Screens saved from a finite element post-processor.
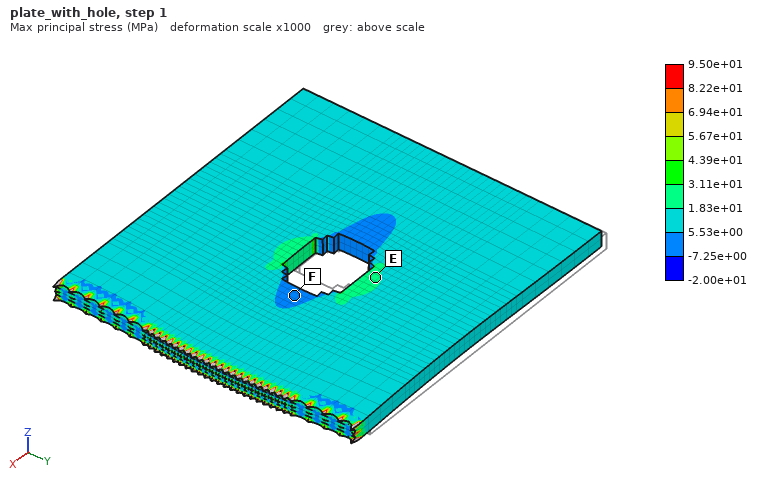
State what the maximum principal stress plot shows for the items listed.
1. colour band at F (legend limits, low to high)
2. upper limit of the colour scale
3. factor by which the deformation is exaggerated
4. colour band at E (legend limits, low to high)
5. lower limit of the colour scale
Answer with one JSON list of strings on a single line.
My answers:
["-7.25e+00 to 5.53e+00 MPa", "9.50e+01 MPa", "1000", "1.83e+01 to 3.11e+01 MPa", "-2.00e+01 MPa"]
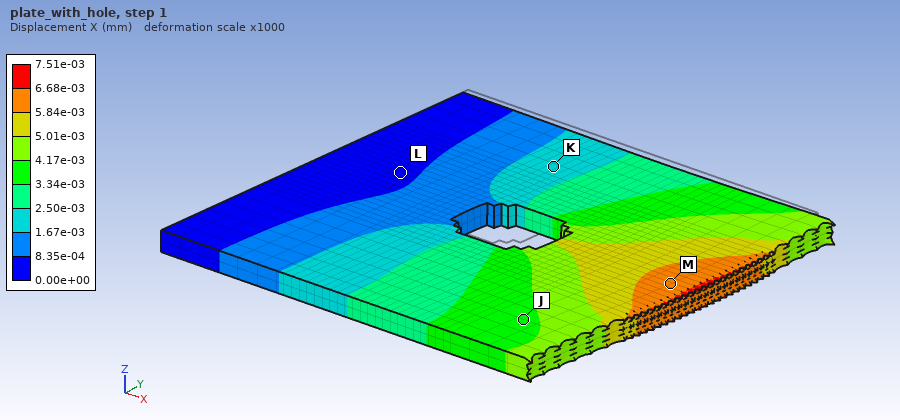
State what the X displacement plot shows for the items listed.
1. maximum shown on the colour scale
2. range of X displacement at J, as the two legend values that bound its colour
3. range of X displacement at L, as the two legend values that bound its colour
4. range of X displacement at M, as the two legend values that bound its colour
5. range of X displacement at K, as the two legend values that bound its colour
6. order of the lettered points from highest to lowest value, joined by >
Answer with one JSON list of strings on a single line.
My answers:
["7.51e-03 mm", "3.34e-03 to 4.17e-03 mm", "0.00e+00 to 8.35e-04 mm", "5.84e-03 to 6.68e-03 mm", "1.67e-03 to 2.50e-03 mm", "M > J > K > L"]
